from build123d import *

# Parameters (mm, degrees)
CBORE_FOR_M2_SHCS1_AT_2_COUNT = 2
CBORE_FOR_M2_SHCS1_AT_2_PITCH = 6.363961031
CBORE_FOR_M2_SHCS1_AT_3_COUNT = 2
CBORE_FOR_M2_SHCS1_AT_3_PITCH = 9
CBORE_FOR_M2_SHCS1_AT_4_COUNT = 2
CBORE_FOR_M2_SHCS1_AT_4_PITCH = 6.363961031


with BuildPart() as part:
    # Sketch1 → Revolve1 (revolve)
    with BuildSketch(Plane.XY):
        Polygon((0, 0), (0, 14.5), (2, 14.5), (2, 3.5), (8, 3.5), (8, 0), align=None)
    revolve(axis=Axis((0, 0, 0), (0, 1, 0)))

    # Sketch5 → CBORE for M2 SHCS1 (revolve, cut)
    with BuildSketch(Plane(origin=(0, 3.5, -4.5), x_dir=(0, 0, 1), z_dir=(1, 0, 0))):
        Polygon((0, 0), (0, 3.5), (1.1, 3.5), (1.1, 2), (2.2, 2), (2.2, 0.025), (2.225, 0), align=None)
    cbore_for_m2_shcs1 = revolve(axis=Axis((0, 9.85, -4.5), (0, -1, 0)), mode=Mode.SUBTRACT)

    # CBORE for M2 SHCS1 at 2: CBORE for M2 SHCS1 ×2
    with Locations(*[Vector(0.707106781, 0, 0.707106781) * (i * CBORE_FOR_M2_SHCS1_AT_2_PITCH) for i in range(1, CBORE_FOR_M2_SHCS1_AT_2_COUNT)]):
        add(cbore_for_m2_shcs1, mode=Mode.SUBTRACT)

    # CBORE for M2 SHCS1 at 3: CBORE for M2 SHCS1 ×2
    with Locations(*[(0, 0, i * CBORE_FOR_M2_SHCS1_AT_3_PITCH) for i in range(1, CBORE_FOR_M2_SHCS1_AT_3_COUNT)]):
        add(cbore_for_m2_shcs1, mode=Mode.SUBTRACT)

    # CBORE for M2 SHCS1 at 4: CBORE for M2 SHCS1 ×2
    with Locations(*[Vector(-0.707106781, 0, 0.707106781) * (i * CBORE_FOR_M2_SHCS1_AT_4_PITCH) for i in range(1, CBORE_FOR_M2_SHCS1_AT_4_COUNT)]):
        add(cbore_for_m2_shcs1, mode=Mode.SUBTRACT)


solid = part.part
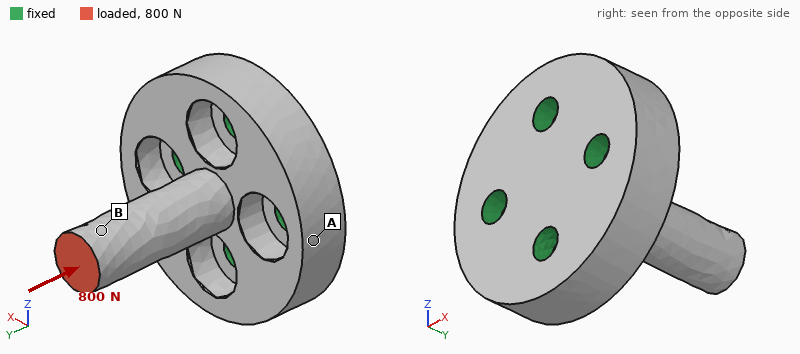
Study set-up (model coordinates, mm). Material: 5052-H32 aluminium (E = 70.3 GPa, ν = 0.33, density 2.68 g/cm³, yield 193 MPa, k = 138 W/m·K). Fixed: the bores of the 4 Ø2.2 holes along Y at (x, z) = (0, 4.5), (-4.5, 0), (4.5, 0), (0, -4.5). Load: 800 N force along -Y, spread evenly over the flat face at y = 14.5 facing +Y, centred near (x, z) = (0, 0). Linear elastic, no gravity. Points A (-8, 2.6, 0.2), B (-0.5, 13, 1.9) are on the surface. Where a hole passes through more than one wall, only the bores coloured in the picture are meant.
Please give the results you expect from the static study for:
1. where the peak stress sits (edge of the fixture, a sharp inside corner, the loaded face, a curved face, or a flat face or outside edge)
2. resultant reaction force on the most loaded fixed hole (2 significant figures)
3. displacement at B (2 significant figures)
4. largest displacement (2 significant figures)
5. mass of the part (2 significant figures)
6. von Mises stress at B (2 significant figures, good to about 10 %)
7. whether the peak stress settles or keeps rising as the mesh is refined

edge of the fixture
220 N
12 µm
14 µm
1.9 g
64 MPa
keeps rising
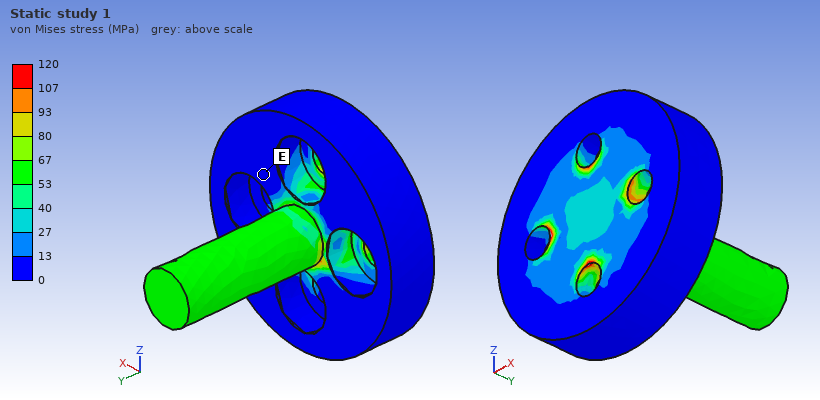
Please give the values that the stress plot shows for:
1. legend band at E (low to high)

0 to 13 MPa
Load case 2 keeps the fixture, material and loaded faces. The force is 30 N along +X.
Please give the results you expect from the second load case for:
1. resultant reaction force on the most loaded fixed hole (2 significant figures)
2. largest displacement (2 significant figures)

46 N
23 µm
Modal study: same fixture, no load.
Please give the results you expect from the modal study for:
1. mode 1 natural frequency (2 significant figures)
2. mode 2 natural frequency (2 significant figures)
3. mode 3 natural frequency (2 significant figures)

18 kHz
18 kHz
66 kHz
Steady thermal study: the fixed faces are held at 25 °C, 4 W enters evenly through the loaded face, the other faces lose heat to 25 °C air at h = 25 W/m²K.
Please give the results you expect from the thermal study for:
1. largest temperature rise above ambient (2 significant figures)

29 K
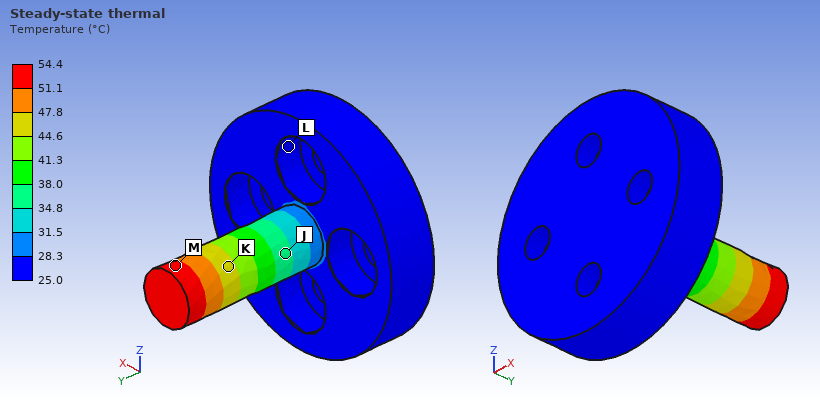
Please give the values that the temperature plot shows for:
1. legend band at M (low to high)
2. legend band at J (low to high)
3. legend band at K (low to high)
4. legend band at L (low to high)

51.1 to 54.4 °C
34.8 to 38.0 °C
44.6 to 47.8 °C
25.0 to 28.3 °C
